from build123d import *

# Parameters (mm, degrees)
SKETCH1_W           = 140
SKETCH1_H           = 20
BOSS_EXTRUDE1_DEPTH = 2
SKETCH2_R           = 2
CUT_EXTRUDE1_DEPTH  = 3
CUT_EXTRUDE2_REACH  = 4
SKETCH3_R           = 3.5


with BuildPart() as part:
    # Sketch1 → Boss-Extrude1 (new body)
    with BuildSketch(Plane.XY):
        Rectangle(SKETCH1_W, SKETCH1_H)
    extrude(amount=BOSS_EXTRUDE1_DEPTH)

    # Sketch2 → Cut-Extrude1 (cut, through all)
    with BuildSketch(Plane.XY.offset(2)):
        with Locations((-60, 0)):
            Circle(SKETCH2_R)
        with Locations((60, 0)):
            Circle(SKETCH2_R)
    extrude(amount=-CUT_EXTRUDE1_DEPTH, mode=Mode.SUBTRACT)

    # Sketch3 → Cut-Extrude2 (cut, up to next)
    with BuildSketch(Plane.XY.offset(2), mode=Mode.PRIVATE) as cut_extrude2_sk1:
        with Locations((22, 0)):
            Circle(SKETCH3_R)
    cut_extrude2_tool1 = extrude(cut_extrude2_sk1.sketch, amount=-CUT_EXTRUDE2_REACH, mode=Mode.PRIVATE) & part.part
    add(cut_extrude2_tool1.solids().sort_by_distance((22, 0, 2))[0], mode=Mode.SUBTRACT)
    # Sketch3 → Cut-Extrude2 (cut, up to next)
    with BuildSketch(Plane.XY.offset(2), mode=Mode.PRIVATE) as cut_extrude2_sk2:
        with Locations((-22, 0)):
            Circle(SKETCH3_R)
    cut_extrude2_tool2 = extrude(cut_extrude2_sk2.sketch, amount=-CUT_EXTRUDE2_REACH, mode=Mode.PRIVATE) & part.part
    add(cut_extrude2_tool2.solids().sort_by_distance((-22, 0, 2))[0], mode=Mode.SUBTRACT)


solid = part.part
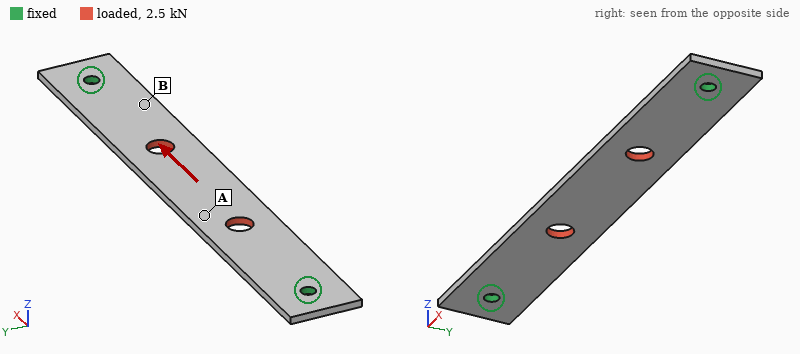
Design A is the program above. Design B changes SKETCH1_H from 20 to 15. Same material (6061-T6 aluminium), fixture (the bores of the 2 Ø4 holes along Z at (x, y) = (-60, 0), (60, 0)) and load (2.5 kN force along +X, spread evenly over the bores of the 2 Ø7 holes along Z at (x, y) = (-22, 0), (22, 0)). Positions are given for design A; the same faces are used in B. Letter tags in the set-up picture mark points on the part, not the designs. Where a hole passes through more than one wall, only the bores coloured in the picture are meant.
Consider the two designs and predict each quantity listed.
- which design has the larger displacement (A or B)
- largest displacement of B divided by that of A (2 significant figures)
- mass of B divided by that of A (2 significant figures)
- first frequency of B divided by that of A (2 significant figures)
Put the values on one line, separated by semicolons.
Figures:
B; 1.3; 0.74; 1.0
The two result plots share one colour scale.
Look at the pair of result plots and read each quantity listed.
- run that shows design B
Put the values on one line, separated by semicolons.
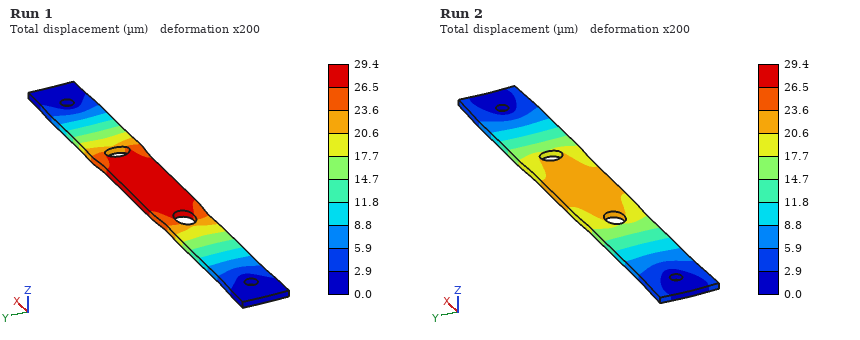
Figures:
Run 1
